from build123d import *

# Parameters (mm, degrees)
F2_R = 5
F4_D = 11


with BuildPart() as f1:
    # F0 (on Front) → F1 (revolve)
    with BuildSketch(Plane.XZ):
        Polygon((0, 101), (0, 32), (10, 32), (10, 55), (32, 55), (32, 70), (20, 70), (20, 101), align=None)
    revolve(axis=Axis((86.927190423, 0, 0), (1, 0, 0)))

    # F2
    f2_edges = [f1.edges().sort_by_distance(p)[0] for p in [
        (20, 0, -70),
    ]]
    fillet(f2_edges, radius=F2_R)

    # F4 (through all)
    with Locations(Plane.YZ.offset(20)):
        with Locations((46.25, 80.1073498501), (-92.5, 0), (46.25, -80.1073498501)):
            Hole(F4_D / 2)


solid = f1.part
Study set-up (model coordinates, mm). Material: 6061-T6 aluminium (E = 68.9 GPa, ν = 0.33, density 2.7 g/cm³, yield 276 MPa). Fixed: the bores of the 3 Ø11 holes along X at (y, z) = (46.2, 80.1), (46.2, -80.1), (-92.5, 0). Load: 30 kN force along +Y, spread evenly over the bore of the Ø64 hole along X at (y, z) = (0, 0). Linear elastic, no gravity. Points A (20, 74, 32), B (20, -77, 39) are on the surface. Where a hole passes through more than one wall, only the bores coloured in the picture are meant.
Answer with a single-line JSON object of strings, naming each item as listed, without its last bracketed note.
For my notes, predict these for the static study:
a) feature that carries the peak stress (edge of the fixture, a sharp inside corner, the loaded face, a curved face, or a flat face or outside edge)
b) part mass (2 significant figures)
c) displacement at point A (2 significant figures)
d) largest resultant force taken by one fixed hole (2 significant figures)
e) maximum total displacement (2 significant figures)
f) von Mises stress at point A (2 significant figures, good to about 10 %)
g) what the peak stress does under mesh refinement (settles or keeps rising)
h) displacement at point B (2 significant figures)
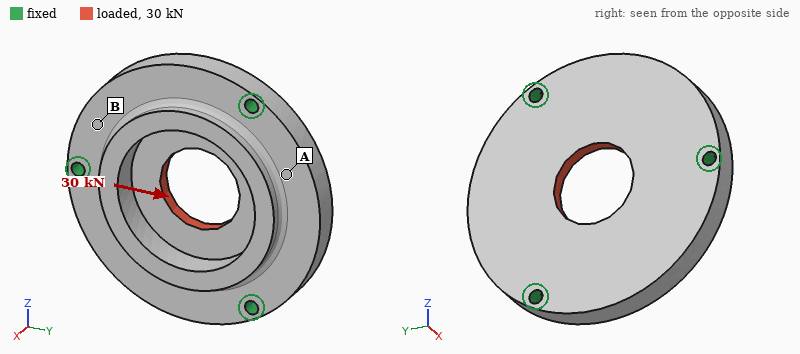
{"feature that carries the peak stress": "edge of the fixture", "part mass": "1.6 kg", "displacement at point A": "14 µm", "largest resultant force taken by one fixed hole": "10 kN", "maximum total displacement": "30 µm", "von Mises stress at point A": "6.9 MPa", "what the peak stress does under mesh refinement": "keeps rising", "displacement at point B": "7.6 µm"}
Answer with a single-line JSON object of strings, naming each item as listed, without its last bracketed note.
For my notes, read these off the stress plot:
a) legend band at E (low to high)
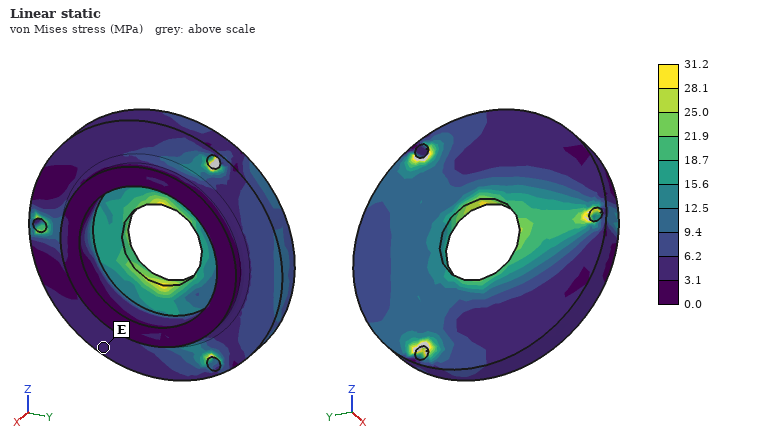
{"legend band at E": "3.1 to 6.2 MPa"}
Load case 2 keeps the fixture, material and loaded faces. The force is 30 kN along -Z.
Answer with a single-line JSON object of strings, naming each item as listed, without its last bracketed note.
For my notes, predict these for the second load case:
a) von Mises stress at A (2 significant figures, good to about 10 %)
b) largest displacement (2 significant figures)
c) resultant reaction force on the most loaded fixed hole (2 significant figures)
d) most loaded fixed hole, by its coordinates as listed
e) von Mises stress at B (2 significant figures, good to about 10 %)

{"von Mises stress at A": "3.5 MPa", "largest displacement": "27 µm", "resultant reaction force on the most loaded fixed hole": "11 kN", "most loaded fixed hole, by its coordinates as listed": "(-92.5, 0)", "von Mises stress at B": "7.7 MPa"}
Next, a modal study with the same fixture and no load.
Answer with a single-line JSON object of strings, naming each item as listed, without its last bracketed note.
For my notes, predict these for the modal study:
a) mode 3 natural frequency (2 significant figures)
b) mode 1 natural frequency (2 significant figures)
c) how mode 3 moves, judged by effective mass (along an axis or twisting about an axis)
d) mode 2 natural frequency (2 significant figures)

{"mode 3 natural frequency": "3300 Hz", "mode 1 natural frequency": "2800 Hz", "how mode 3 moves, judged by effective mass": "along X", "mode 2 natural frequency": "2800 Hz"}
